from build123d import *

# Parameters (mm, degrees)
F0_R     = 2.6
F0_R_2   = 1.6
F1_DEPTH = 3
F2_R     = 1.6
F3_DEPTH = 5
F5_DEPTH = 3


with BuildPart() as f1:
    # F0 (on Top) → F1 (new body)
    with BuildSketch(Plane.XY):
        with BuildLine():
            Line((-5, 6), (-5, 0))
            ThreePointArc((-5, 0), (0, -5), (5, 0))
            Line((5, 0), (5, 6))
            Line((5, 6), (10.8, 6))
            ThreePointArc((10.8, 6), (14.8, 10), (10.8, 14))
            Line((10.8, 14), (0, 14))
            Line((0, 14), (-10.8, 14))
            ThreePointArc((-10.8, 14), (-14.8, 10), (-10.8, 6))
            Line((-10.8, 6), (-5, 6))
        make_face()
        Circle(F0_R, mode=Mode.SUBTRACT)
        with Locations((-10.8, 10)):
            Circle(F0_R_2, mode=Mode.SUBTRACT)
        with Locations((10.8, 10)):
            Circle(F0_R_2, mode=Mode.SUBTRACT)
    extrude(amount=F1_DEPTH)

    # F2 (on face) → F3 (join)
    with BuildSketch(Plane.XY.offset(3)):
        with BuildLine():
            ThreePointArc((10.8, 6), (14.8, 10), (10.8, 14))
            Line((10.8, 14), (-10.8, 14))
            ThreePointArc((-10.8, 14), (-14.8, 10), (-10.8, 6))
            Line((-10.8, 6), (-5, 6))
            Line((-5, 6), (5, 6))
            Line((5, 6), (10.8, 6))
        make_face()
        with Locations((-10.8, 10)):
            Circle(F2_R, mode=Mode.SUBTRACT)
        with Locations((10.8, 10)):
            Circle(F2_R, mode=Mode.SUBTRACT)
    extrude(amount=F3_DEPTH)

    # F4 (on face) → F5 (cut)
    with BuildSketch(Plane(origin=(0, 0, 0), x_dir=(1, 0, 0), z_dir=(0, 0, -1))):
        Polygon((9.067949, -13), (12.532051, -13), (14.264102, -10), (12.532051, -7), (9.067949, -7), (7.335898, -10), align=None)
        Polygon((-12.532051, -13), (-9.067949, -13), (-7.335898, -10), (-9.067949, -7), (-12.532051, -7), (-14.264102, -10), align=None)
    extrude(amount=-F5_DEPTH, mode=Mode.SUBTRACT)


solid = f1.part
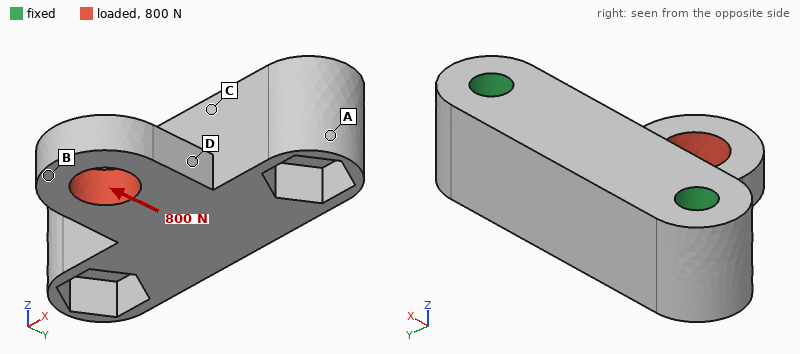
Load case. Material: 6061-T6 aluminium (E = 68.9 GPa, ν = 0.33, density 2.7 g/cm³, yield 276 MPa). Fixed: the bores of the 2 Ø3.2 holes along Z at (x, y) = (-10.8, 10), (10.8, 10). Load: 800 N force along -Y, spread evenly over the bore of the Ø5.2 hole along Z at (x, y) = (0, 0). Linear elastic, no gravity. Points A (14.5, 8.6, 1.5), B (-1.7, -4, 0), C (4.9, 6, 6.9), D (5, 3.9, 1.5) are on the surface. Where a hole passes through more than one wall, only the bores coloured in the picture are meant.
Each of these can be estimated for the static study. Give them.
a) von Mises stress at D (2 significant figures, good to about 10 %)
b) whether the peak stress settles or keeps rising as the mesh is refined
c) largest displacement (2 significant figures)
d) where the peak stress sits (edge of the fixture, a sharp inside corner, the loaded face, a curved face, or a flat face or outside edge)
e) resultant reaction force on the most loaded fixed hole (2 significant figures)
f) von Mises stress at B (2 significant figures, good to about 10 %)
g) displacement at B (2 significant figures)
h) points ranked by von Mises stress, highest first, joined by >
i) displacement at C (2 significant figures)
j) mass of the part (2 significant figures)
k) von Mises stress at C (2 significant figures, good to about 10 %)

42 MPa
keeps rising
26 µm
edge of the fixture
400 N
26 MPa
24 µm
D > B > C > A
3.9 µm
4.7 g
16 MPa
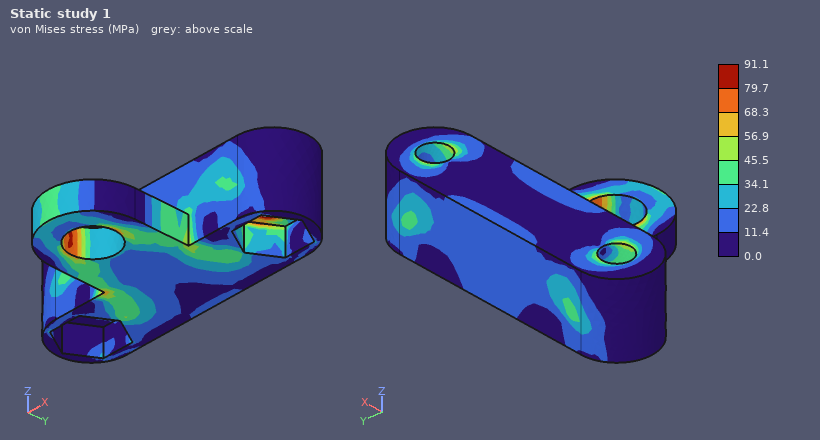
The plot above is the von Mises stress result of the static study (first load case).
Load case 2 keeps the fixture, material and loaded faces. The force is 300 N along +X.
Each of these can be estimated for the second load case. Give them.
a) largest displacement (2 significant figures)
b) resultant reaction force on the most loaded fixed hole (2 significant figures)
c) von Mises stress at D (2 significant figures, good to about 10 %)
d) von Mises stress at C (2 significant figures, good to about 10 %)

18 µm
220 N
42 MPa
7.7 MPa
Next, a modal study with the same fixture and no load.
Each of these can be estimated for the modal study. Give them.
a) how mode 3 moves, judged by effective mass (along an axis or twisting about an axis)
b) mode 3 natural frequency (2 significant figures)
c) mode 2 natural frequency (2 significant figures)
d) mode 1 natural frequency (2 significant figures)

along Y
36 kHz
33 kHz
16 kHz
